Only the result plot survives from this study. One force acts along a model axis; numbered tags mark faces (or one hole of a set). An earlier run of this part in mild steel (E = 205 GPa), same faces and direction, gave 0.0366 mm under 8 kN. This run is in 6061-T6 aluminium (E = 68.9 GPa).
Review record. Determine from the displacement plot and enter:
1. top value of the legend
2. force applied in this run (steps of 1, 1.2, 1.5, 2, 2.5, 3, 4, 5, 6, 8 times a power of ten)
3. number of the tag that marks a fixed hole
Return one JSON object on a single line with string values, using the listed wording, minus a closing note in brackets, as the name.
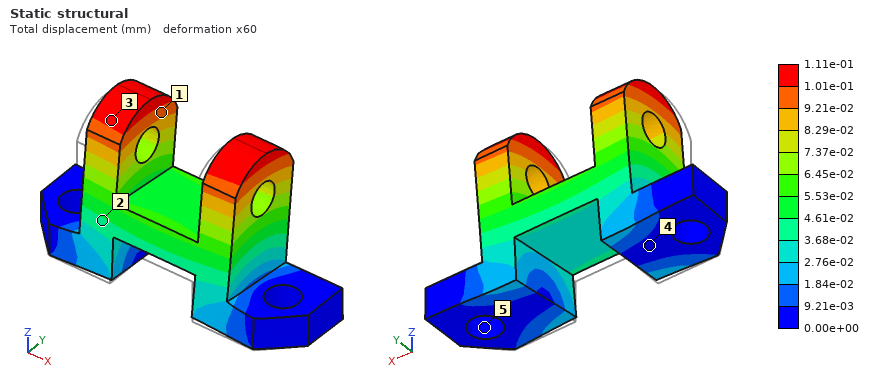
{"top value of the legend": "1.11e-01 mm", "force applied in this run": "8 kN", "number of the tag that marks a fixed hole": "5"}
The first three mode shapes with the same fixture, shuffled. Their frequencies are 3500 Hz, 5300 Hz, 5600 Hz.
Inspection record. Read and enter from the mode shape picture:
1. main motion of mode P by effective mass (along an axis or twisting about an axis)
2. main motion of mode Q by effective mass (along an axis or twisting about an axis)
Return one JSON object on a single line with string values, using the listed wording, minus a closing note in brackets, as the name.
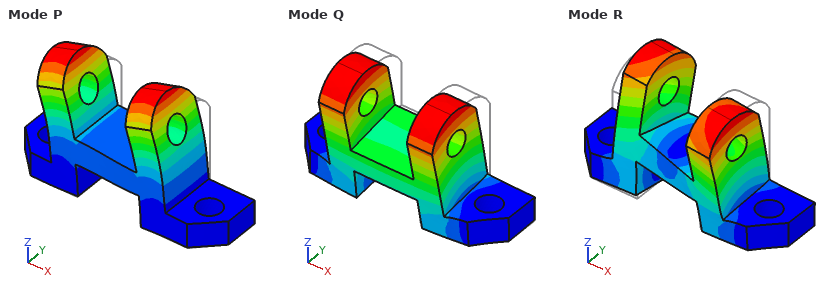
{"main motion of mode P by effective mass": "along X", "main motion of mode Q by effective mass": "along Y"}
